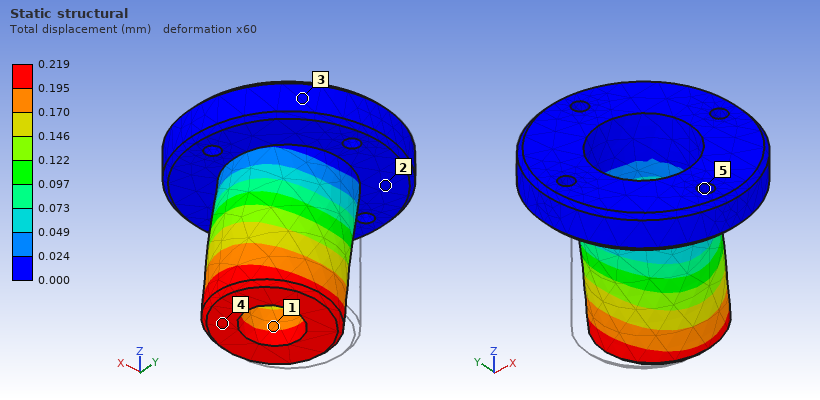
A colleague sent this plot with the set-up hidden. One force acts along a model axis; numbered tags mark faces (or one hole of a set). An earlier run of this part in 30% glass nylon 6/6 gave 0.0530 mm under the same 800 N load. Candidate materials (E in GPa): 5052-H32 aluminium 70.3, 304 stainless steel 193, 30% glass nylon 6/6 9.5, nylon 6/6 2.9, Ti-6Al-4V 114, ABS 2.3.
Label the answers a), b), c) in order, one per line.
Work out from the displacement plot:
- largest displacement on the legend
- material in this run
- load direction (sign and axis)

a) 0.219 mm
b) ABS
c) +X
